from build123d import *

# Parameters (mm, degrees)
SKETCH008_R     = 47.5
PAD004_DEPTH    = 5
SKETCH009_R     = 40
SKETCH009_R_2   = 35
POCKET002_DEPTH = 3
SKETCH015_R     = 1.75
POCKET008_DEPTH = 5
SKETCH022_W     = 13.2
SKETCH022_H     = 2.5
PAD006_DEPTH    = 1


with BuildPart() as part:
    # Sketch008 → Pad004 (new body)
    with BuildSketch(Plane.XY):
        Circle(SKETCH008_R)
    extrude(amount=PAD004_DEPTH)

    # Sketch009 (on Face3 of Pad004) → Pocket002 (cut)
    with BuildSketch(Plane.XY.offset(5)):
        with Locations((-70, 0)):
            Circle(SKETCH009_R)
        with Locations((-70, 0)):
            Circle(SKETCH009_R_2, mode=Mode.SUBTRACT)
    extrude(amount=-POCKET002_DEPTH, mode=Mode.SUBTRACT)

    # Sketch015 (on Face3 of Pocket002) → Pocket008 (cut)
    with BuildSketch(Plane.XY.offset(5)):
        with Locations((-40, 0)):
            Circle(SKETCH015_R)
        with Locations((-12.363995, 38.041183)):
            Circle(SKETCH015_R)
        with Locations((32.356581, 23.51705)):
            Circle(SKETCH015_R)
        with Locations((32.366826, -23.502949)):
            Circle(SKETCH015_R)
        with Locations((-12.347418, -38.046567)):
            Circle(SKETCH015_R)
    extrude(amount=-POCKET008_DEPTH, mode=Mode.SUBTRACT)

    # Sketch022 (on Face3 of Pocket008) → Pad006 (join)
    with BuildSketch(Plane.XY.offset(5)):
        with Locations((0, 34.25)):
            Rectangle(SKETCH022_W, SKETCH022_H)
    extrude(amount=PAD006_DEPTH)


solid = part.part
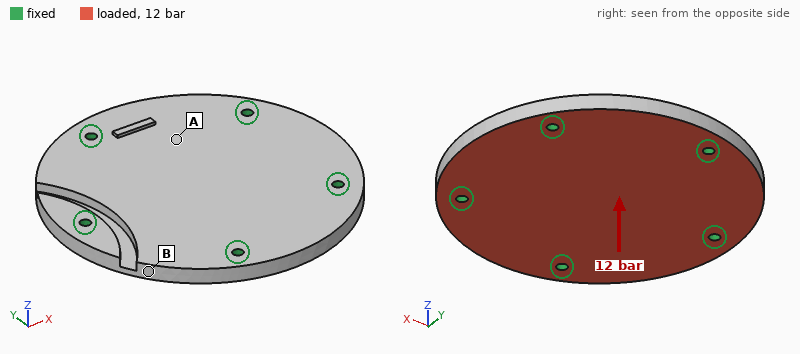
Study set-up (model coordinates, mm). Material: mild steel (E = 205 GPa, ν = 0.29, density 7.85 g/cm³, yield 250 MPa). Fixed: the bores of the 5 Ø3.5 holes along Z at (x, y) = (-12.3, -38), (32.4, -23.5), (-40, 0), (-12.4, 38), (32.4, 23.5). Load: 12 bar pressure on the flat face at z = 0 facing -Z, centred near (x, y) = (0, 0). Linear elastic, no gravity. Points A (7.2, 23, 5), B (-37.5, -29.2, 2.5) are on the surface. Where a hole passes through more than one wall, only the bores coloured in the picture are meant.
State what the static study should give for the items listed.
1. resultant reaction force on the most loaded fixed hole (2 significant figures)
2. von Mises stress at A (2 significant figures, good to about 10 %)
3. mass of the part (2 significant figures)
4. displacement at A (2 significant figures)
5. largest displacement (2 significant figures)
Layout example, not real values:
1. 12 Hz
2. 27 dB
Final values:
1. 1.7 kN
2. 37 MPa
3. 270 g
4. 21 µm
5. 37 µm
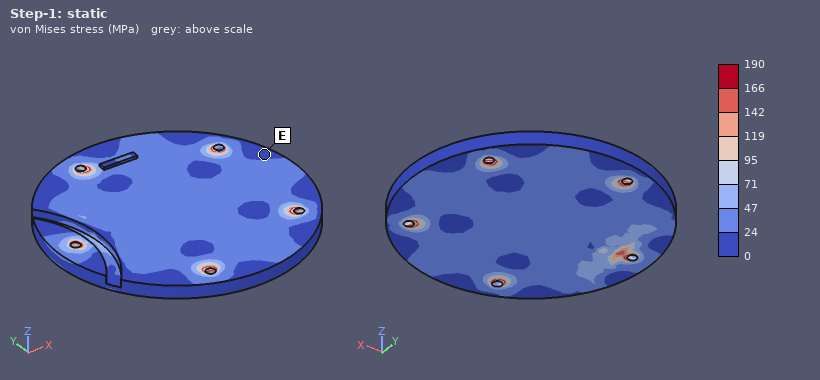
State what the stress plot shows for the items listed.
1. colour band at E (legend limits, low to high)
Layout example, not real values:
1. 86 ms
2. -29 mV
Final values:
1. 0 to 24 MPa
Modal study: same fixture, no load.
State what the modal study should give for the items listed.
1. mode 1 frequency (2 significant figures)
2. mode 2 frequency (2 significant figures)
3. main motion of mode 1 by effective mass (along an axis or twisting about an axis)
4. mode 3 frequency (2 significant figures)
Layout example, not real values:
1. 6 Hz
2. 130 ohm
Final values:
1. 5600 Hz
2. 8700 Hz
3. along Z
4. 8700 Hz
